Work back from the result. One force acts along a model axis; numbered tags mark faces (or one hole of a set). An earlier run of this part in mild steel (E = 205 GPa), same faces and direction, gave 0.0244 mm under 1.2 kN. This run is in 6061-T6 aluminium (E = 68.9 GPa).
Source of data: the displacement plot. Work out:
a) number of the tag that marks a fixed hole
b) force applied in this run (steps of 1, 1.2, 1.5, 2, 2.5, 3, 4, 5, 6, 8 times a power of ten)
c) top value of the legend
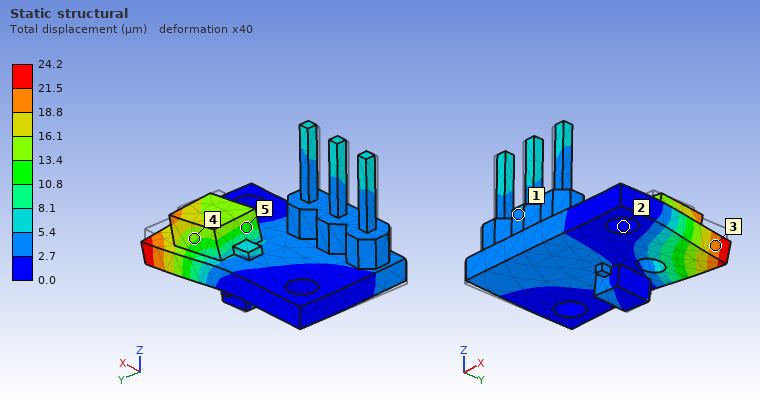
2
400 N
24.2 µm
